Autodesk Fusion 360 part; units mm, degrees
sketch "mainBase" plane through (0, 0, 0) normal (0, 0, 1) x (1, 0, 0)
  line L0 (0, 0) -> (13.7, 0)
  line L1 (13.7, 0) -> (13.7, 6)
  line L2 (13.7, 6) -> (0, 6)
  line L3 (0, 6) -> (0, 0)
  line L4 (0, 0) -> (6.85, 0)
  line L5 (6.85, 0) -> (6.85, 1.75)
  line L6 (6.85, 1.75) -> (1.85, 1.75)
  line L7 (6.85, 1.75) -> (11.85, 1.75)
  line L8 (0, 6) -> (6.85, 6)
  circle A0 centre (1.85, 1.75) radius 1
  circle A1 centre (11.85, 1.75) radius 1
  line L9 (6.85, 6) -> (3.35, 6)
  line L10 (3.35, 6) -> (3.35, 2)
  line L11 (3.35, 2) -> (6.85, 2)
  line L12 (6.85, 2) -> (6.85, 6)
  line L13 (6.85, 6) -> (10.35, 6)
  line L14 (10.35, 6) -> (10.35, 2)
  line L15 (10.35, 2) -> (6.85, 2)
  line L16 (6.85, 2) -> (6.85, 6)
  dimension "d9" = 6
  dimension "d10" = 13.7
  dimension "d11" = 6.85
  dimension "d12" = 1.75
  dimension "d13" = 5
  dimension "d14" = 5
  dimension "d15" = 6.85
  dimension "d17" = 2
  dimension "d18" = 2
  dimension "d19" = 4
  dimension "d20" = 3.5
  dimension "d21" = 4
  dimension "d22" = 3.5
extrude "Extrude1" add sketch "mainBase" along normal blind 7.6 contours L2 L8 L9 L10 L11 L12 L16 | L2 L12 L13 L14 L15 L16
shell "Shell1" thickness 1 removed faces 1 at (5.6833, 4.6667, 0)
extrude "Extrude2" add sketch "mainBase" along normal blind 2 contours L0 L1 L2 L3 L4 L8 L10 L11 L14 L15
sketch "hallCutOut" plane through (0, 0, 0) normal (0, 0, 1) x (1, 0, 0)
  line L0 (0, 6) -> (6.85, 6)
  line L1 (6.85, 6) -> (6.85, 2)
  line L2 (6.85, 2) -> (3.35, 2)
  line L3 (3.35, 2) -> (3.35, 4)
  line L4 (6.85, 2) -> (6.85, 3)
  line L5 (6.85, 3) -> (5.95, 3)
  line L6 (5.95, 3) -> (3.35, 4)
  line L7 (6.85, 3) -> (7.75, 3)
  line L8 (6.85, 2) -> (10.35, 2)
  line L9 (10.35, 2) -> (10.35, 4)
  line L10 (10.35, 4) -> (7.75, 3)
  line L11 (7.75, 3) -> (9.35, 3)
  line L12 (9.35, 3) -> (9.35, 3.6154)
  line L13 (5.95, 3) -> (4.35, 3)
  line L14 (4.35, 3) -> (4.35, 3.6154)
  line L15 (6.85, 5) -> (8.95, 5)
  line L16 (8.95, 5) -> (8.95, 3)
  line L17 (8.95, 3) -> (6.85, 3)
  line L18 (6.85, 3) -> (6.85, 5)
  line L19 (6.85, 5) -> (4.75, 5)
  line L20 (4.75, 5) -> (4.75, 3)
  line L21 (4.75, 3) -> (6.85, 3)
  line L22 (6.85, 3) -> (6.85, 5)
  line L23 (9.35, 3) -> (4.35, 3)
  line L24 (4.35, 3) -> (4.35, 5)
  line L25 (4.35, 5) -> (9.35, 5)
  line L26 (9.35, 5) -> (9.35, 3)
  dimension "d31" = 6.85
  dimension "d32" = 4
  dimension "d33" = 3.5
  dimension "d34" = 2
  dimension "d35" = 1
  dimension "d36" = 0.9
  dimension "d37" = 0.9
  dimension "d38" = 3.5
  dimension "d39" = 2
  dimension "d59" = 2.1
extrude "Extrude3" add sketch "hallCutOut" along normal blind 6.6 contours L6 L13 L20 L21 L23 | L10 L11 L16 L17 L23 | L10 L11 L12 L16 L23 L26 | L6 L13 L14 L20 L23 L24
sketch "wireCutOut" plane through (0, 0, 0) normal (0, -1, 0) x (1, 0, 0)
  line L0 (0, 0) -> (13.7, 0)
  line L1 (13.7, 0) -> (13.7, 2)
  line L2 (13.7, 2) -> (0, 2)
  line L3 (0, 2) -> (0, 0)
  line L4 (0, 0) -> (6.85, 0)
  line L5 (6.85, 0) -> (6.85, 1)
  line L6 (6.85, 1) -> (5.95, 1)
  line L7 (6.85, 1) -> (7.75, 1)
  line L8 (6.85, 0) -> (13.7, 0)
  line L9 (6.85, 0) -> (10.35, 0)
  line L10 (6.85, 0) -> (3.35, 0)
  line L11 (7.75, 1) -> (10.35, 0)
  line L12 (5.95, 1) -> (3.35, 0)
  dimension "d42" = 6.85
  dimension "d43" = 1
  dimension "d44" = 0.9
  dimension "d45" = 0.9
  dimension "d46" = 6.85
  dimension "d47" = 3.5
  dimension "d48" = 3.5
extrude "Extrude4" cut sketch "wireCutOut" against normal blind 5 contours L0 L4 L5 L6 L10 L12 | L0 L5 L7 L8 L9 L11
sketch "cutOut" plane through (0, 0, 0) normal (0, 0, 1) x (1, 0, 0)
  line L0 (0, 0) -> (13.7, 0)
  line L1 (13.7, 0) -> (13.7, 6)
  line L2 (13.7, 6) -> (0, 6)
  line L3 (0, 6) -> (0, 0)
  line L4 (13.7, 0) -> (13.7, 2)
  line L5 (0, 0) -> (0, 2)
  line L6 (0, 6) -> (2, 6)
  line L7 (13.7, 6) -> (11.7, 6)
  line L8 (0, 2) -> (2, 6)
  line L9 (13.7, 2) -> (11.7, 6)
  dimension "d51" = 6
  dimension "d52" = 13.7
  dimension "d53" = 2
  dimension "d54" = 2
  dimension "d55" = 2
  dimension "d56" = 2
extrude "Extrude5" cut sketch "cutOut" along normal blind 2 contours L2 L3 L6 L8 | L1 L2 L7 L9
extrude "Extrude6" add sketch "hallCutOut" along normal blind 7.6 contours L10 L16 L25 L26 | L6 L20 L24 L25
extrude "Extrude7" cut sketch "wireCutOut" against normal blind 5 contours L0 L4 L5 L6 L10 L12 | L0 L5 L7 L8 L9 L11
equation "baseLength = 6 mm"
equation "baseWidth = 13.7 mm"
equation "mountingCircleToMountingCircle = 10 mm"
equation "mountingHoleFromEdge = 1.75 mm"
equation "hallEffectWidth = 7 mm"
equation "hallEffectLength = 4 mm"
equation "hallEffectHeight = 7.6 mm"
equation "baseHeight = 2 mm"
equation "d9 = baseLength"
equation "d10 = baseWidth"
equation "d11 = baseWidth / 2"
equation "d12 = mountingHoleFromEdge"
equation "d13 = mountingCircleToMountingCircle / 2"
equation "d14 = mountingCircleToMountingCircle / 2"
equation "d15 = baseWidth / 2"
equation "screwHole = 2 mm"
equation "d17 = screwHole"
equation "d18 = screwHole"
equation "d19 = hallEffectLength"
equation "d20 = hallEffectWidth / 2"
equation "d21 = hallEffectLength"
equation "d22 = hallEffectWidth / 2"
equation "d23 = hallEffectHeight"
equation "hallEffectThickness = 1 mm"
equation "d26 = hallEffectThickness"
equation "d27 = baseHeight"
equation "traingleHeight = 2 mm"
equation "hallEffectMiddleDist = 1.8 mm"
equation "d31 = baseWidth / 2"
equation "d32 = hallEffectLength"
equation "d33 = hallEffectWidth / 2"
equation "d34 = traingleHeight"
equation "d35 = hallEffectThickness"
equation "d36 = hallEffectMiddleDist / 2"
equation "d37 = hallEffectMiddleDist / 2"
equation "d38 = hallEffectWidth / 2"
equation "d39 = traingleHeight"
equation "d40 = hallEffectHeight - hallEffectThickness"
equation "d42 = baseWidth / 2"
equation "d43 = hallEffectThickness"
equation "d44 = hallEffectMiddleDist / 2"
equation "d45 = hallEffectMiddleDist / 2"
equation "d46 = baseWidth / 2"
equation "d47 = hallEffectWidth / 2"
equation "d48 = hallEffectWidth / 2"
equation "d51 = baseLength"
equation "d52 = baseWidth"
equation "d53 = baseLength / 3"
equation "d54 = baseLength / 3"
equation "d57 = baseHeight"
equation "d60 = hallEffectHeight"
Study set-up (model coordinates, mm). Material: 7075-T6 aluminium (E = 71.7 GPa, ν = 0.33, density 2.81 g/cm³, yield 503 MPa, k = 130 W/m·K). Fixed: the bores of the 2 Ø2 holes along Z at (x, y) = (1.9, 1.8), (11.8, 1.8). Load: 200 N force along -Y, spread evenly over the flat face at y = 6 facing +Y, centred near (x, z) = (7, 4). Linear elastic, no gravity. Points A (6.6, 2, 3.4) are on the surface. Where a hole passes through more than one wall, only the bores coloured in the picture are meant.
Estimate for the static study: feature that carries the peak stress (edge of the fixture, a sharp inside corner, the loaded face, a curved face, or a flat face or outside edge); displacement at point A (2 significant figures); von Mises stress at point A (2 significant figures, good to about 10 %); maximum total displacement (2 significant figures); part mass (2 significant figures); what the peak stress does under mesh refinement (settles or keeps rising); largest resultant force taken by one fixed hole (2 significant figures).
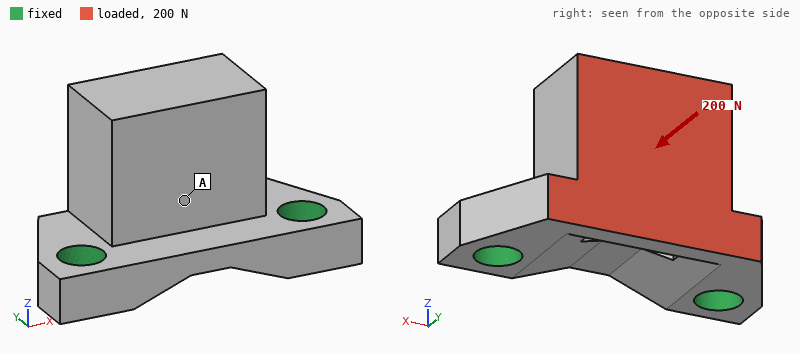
a sharp inside corner
6.1 µm
16 MPa
20 µm
0.63 g
keeps rising
110 N
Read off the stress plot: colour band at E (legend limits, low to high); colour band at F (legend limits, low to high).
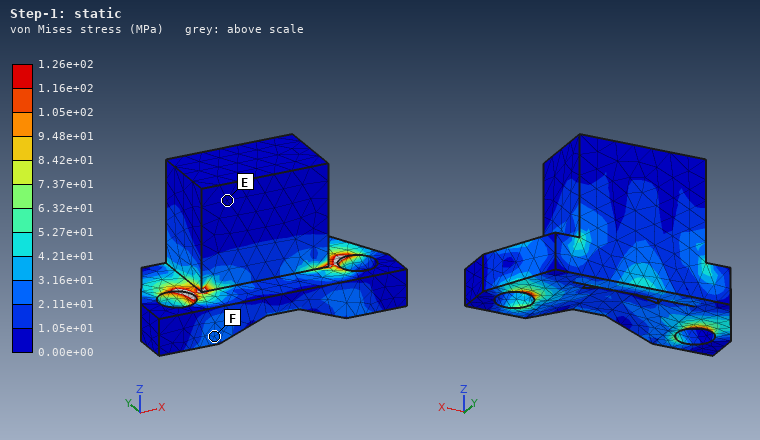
0.00e+00 to 1.05e+01 MPa
2.11e+01 to 3.16e+01 MPa
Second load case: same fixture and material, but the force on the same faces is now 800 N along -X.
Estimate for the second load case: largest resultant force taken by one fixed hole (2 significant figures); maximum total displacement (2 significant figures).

530 N
22 µm
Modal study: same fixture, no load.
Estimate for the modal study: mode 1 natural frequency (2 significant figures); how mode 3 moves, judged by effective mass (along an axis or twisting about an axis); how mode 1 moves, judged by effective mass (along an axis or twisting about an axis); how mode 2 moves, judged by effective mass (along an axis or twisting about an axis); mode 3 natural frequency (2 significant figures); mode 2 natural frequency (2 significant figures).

25 kHz
along Z
along Y
along X
75 kHz
56 kHz
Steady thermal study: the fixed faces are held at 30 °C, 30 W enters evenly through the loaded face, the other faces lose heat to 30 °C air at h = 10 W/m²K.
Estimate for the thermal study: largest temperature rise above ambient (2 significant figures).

68 K
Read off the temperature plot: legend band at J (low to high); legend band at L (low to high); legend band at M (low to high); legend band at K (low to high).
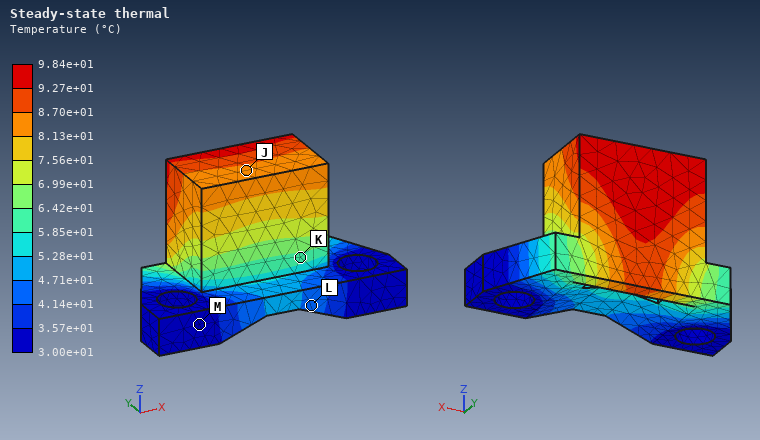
8.13e+01 to 8.70e+01 °C
4.14e+01 to 4.71e+01 °C
3.00e+01 to 3.57e+01 °C
5.85e+01 to 6.42e+01 °C
